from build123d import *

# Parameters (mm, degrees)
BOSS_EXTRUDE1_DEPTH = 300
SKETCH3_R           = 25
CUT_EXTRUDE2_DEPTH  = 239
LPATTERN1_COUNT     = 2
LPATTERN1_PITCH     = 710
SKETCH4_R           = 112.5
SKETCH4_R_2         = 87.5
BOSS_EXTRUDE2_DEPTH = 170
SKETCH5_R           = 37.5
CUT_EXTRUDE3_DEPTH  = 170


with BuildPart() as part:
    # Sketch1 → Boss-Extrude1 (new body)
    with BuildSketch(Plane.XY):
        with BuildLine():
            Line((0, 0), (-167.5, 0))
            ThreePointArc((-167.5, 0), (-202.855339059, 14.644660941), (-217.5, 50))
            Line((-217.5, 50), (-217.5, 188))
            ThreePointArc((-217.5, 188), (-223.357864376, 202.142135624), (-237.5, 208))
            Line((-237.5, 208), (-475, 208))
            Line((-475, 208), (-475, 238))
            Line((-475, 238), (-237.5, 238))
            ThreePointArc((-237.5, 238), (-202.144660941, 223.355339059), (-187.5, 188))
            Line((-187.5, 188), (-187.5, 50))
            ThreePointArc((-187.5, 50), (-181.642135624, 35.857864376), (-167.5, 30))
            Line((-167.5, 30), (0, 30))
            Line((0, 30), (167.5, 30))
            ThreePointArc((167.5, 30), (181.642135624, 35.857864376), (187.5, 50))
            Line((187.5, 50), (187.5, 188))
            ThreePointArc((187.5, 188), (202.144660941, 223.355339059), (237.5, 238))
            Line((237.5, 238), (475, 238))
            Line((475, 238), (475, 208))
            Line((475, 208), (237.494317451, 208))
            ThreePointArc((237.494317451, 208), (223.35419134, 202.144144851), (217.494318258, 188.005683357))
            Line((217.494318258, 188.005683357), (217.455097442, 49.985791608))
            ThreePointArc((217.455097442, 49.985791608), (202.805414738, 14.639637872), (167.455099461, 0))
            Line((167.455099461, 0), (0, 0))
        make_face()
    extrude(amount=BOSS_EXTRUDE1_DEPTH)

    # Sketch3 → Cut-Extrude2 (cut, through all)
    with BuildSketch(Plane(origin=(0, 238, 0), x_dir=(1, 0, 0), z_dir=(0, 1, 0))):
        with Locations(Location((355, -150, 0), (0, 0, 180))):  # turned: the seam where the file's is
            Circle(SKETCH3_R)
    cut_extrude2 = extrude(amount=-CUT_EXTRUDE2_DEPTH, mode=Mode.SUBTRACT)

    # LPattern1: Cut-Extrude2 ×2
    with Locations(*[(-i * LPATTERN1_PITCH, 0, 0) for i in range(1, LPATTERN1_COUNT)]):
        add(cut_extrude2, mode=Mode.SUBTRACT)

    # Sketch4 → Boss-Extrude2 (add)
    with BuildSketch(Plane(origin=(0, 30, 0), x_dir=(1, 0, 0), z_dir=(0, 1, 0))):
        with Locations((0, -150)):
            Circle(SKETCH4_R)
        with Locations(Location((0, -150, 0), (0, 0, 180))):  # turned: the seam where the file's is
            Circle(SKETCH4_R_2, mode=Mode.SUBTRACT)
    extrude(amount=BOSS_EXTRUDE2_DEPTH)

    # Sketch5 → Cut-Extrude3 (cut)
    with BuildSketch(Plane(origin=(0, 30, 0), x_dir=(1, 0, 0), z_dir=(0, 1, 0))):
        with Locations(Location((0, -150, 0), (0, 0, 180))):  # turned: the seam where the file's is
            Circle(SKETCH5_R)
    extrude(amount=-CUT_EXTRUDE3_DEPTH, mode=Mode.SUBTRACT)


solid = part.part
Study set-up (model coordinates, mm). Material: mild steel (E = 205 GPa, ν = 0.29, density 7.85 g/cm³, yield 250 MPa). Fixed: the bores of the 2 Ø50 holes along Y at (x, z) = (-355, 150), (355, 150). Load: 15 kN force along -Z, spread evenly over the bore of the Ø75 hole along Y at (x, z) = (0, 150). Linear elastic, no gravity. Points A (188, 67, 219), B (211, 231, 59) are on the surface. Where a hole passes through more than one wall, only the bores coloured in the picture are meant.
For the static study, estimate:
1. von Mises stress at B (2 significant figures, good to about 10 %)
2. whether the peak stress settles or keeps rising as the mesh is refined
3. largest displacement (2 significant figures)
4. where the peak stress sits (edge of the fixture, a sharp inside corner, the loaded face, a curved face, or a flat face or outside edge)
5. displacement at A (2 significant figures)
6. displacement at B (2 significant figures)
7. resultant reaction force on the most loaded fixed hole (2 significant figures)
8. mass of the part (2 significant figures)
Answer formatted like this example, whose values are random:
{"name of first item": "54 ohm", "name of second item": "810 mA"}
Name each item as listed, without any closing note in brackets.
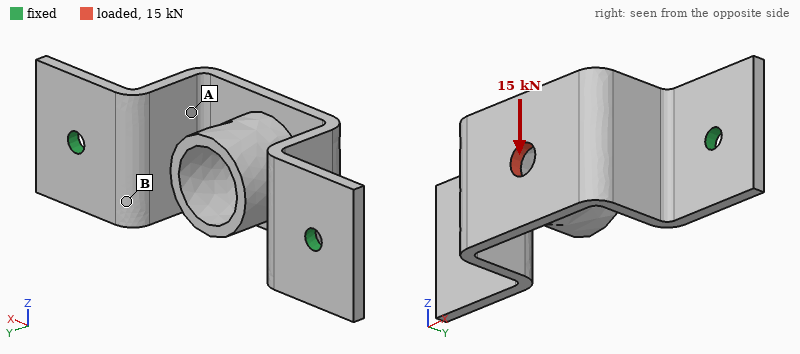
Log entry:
{"von Mises stress at B": "12 MPa", "whether the peak stress settles or keeps rising as the mesh is refined": "keeps rising", "largest displacement": "0.24 mm", "where the peak stress sits": "edge of the fixture", "displacement at A": "0.16 mm", "displacement at B": "0.076 mm", "resultant reaction force on the most loaded fixed hole": "7.5 kN", "mass of the part": "110 kg"}
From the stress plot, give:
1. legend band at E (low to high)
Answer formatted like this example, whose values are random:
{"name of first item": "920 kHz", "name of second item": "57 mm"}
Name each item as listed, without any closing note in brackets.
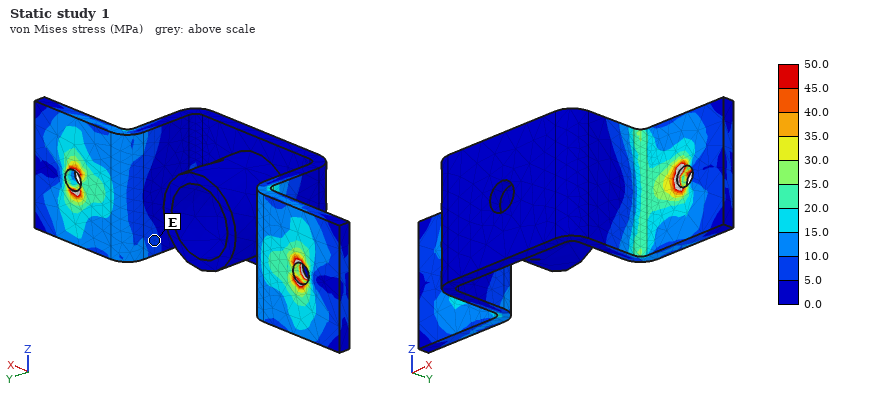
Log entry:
{"legend band at E": "5.0 to 10.0 MPa"}
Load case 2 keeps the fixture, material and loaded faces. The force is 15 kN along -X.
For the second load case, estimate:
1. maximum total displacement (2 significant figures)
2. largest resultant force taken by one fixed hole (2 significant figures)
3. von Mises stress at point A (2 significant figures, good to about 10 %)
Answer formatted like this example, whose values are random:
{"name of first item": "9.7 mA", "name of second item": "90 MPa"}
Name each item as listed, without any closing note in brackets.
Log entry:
{"maximum total displacement": "0.14 mm", "largest resultant force taken by one fixed hole": "8.6 kN", "von Mises stress at point A": "10 MPa"}
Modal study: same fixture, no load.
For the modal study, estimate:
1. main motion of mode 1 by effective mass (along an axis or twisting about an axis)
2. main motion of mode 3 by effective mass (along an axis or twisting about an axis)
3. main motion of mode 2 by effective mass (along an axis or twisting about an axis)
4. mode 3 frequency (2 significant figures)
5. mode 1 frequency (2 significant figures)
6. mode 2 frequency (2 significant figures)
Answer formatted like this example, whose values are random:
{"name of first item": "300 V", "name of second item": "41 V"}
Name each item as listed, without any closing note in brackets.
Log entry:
{"main motion of mode 1 by effective mass": "along Z", "main motion of mode 3 by effective mass": "along Y", "main motion of mode 2 by effective mass": "along X", "mode 3 frequency": "390 Hz", "mode 1 frequency": "190 Hz", "mode 2 frequency": "230 Hz"}
